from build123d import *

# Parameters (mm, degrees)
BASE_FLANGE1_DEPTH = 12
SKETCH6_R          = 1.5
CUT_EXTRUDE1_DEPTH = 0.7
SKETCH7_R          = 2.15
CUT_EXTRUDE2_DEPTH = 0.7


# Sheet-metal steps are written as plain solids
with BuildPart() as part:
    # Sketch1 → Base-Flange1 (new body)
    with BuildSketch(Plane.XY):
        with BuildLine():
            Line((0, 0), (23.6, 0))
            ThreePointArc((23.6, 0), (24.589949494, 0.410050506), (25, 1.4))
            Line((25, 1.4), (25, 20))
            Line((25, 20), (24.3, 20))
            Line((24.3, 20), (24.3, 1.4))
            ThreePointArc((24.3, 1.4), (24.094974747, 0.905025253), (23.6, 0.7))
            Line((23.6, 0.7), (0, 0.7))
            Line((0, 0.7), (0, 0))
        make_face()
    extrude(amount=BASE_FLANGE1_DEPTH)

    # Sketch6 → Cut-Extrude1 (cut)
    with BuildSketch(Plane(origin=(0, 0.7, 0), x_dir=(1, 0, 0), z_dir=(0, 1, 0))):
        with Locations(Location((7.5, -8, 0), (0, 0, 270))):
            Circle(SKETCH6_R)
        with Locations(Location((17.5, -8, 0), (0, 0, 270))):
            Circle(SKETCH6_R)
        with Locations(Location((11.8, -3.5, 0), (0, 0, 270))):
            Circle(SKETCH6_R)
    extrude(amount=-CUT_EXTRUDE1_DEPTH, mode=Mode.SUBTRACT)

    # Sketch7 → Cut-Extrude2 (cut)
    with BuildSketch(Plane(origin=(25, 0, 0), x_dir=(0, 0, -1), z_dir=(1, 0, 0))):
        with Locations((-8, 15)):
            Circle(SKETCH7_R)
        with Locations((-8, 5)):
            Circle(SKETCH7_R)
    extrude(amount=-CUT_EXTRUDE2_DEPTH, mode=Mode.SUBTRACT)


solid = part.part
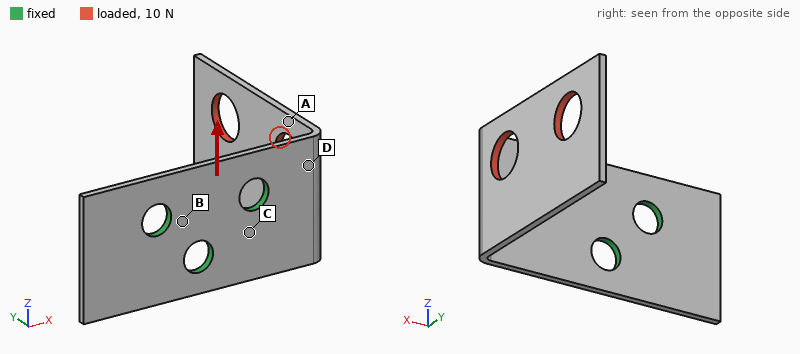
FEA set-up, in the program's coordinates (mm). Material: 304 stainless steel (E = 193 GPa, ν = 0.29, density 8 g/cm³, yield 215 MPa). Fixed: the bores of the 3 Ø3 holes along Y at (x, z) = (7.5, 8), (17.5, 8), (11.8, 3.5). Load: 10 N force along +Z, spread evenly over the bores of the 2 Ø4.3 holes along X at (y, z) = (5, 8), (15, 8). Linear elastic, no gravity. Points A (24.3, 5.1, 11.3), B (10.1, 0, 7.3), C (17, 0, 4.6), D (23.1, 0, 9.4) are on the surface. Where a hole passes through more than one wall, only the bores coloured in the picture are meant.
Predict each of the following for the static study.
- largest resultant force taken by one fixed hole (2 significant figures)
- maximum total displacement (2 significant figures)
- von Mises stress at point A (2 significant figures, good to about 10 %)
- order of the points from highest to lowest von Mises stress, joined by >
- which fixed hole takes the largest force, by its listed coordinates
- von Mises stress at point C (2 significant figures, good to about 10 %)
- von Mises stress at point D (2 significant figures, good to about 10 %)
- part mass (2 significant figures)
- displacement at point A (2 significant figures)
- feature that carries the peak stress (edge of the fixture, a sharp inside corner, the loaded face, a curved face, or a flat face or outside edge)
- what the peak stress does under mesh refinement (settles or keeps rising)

13 N
0.10 mm
29 MPa
D > C > A > B
(17.5, 8)
51 MPa
64 MPa
2.7 g
0.028 mm
edge of the fixture
keeps rising
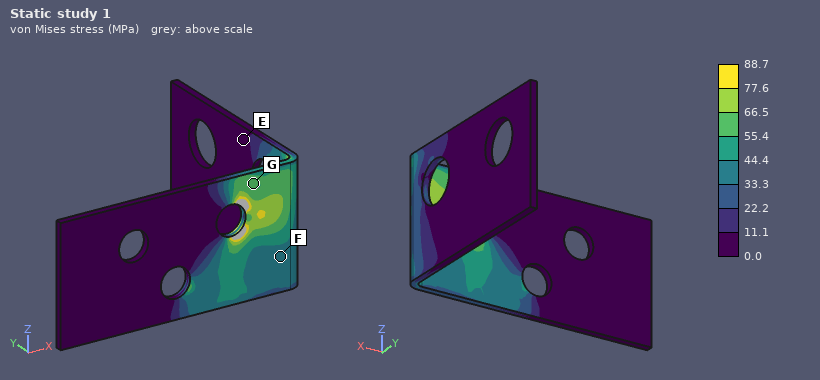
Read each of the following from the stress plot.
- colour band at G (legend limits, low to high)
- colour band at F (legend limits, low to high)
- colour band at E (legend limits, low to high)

55.4 to 66.5 MPa
33.3 to 44.4 MPa
0.0 to 11.1 MPa
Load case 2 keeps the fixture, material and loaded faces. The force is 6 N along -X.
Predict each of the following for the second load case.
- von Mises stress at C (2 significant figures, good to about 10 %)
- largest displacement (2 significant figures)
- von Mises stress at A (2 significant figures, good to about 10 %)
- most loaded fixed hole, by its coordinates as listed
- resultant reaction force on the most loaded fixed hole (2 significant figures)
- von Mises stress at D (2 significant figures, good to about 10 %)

17 MPa
0.21 mm
58 MPa
(17.5, 8)
5.8 N
55 MPa
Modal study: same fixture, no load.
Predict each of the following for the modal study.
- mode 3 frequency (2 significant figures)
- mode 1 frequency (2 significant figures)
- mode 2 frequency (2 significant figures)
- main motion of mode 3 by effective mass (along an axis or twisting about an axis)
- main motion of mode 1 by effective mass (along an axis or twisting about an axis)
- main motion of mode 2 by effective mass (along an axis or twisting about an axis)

4500 Hz
970 Hz
1800 Hz
along Y
along X
along Z
